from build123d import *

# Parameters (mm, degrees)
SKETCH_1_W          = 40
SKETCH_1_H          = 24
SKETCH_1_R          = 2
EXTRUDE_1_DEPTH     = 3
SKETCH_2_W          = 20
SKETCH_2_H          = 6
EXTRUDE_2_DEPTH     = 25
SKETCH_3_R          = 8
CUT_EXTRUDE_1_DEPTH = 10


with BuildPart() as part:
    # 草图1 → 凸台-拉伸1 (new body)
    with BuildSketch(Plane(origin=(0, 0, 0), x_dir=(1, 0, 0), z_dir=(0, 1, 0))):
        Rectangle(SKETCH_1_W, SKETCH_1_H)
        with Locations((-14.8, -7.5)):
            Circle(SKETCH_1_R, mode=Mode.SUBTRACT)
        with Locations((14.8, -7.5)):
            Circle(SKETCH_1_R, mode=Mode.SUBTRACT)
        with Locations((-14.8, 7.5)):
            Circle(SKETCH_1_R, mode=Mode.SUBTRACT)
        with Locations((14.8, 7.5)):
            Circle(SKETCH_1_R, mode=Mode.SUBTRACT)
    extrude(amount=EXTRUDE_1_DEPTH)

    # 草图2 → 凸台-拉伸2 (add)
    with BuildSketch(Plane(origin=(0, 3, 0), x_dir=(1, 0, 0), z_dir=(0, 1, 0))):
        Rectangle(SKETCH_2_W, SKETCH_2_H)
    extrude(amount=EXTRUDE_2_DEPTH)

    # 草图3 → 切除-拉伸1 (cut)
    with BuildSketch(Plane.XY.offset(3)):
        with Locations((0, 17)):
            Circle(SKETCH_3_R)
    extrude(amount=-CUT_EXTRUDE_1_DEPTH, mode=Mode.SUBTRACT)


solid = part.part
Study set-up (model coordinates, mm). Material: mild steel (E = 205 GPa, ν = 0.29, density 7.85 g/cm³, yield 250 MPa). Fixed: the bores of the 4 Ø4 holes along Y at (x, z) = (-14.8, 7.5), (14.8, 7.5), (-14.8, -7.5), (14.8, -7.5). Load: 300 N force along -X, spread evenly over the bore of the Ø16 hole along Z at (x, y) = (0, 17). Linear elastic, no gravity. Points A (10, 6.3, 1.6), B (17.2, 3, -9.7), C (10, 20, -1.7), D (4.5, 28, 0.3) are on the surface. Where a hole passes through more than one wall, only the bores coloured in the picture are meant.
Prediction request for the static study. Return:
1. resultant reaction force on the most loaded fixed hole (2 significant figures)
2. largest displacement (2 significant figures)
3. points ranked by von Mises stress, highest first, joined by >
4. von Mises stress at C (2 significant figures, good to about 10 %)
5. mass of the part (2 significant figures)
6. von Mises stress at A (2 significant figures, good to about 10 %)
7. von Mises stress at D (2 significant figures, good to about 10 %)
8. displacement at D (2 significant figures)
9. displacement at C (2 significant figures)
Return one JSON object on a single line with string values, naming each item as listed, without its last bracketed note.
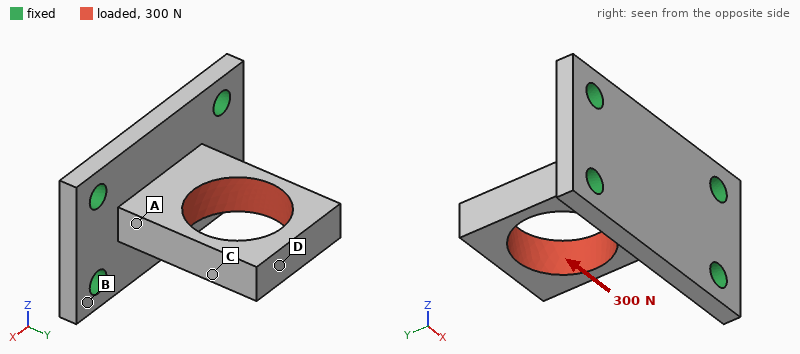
{"resultant reaction force on the most loaded fixed hole": "130 N", "largest displacement": "12 µm", "points ranked by von Mises stress, highest first, joined by >": "C > A > D > B", "von Mises stress at C": "28 MPa", "mass of the part": "36 g", "von Mises stress at A": "19 MPa", "von Mises stress at D": "12 MPa", "displacement at D": "12 µm", "displacement at C": "9.5 µm"}
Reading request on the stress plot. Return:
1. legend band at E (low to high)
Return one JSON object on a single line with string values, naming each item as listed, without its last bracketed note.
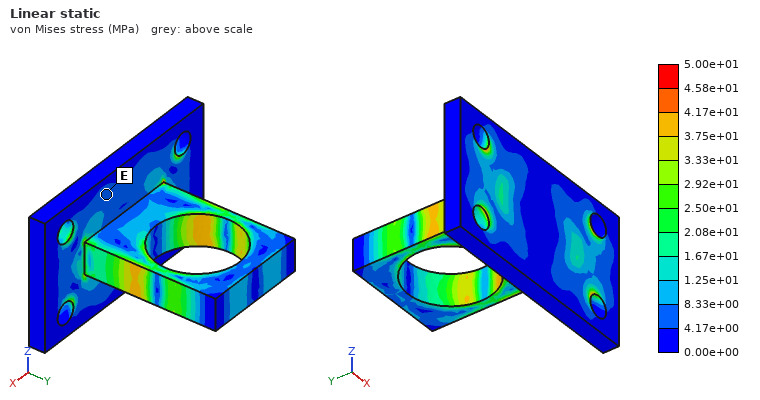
{"legend band at E": "4.17e+00 to 8.33e+00 MPa"}
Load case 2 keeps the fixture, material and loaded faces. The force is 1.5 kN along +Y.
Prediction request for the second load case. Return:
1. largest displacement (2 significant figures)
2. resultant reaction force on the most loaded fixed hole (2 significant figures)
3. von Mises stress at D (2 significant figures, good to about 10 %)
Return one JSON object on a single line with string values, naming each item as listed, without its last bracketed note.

{"largest displacement": "12 µm", "resultant reaction force on the most loaded fixed hole": "390 N", "von Mises stress at D": "22 MPa"}
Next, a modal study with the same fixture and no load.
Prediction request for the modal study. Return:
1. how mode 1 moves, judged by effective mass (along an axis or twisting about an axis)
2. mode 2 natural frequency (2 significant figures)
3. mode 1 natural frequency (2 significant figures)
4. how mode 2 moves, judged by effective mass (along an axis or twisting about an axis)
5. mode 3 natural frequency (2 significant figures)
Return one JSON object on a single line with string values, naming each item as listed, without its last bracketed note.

{"how mode 1 moves, judged by effective mass": "along Z", "mode 2 natural frequency": "8200 Hz", "mode 1 natural frequency": "5100 Hz", "how mode 2 moves, judged by effective mass": "along X", "mode 3 natural frequency": "12 kHz"}
